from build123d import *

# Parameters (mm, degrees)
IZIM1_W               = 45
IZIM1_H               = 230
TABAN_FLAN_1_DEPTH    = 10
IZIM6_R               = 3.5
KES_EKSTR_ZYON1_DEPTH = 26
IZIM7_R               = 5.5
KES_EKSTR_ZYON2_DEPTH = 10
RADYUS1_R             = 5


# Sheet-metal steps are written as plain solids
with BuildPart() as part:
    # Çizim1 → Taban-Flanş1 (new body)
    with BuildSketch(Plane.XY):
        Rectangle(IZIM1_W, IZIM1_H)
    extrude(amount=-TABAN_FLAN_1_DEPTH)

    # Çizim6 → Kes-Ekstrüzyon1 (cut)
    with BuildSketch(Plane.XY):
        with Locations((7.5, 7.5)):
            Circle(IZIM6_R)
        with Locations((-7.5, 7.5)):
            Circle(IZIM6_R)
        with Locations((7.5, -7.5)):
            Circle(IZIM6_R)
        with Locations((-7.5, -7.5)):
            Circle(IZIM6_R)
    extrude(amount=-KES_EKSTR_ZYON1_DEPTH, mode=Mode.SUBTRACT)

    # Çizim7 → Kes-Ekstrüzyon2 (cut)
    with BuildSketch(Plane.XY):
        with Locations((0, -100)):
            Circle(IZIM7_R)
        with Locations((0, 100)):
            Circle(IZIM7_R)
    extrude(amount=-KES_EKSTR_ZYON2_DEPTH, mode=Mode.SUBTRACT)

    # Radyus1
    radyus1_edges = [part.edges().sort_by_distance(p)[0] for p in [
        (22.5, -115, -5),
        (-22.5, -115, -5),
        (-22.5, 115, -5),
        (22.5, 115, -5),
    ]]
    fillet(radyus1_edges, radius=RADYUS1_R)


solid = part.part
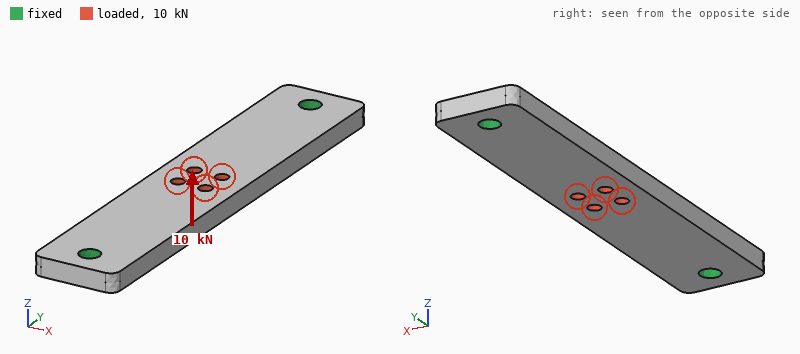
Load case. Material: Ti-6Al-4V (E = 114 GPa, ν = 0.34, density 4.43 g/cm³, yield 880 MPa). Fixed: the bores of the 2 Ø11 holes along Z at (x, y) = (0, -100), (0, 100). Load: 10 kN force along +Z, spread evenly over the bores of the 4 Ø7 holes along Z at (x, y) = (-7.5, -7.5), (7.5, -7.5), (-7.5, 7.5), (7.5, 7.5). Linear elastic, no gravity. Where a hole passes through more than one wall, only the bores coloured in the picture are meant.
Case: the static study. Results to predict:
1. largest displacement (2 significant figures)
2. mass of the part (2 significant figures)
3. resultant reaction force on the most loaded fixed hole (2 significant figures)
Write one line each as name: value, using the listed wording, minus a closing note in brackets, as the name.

largest displacement: 1.0 mm
mass of the part: 440 g
resultant reaction force on the most loaded fixed hole: 5.0 kN
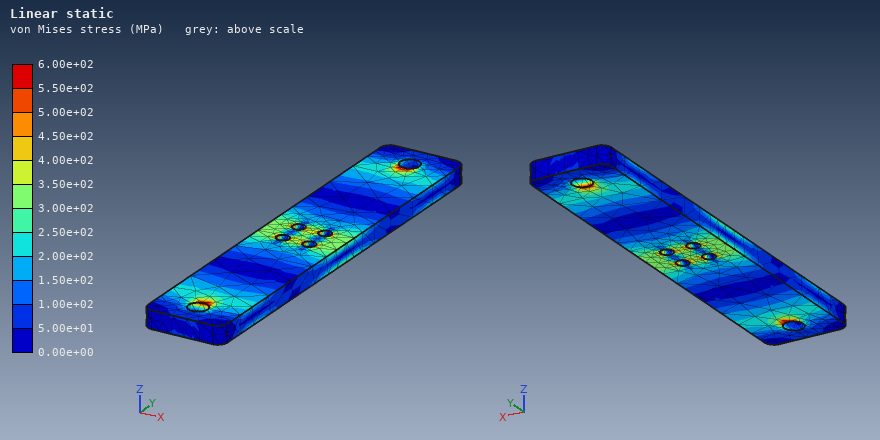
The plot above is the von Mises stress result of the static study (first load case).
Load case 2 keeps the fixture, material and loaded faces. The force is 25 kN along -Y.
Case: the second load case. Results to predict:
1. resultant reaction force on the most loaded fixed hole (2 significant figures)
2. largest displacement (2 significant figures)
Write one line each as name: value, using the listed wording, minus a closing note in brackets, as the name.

resultant reaction force on the most loaded fixed hole: 13 kN
largest displacement: 29 µm
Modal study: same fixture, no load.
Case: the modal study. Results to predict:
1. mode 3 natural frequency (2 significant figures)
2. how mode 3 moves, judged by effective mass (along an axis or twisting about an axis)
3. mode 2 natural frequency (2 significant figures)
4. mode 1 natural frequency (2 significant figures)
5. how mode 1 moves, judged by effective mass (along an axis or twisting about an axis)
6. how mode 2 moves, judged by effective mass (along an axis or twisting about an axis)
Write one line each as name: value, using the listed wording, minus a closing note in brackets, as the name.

mode 3 natural frequency: 3500 Hz
how mode 3 moves, judged by effective mass: along X
mode 2 natural frequency: 3300 Hz
mode 1 natural frequency: 1300 Hz
how mode 1 moves, judged by effective mass: along Z
how mode 2 moves, judged by effective mass: twisting about Y
